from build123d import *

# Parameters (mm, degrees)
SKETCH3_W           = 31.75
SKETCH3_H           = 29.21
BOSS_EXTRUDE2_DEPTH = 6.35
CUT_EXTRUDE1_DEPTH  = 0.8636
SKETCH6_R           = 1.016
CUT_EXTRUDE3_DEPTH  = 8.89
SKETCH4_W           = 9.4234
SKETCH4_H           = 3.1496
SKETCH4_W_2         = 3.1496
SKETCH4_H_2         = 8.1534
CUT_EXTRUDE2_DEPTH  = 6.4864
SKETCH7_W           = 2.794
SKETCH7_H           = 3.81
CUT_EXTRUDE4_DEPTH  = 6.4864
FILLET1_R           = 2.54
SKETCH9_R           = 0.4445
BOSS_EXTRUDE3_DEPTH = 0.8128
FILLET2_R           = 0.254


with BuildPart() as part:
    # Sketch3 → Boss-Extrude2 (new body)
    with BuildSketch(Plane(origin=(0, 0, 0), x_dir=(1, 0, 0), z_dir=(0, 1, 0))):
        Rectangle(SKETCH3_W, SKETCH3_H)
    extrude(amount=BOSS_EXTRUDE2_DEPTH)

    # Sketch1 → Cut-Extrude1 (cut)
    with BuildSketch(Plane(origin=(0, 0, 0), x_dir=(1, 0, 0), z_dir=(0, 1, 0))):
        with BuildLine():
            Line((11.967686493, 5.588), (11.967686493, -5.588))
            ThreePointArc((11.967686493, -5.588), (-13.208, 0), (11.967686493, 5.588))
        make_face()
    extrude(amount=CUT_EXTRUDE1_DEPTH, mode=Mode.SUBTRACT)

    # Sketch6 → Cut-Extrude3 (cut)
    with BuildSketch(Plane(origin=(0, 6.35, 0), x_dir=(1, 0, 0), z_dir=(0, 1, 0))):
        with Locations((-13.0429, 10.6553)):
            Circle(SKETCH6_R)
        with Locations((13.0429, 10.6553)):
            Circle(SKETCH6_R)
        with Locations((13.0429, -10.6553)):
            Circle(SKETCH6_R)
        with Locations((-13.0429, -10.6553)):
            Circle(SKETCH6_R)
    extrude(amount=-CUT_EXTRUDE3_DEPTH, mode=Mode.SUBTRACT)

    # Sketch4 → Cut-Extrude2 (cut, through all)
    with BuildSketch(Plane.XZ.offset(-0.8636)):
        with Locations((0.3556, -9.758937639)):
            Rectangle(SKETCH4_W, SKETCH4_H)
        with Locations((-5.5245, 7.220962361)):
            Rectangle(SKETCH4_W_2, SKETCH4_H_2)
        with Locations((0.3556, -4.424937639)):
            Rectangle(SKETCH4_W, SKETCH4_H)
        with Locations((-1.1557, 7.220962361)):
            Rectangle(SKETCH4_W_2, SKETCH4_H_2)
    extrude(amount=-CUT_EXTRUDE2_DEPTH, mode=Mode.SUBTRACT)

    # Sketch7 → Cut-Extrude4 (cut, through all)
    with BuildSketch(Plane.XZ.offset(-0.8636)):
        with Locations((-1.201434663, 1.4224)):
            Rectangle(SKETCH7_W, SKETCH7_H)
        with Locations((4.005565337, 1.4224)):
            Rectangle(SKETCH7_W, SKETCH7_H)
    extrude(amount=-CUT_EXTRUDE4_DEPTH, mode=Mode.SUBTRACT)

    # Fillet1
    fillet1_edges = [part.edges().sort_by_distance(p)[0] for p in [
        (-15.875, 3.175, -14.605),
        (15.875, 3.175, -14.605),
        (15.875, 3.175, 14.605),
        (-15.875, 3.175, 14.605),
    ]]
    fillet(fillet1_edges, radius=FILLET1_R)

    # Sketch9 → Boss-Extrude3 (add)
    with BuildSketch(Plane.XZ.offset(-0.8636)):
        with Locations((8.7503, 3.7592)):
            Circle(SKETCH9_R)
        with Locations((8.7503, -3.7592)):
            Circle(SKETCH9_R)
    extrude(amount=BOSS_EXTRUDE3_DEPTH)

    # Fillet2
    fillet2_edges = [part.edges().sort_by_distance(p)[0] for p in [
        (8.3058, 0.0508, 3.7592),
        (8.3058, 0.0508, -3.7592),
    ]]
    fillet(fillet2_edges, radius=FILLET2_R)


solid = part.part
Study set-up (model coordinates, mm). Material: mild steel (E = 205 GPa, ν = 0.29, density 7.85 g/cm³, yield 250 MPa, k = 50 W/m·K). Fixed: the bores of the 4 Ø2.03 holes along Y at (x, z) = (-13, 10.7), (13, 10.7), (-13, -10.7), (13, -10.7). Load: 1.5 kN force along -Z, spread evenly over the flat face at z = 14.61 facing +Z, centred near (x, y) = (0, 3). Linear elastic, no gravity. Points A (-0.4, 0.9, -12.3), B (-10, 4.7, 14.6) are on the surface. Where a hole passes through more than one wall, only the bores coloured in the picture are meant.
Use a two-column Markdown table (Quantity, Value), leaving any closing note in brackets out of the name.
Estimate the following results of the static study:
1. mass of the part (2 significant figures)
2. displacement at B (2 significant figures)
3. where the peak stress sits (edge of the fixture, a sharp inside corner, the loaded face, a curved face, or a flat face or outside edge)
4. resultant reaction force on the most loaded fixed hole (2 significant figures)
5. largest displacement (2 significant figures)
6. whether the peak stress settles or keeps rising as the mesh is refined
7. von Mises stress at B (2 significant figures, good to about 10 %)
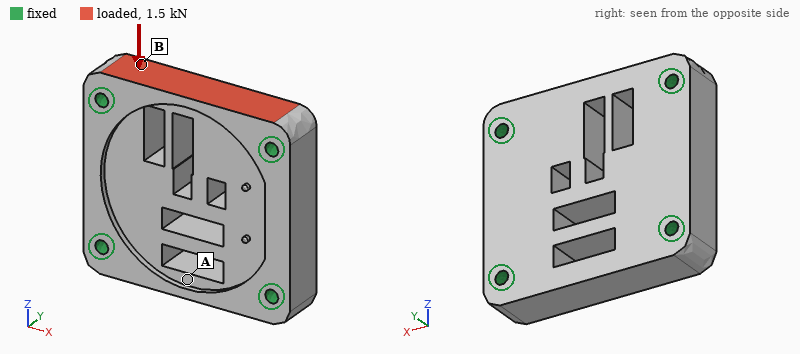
| Quantity | Value |
|---|---|
| mass of the part | 36 g |
| displacement at B | 0.61 µm |
| where the peak stress sits | a sharp inside corner |
| resultant reaction force on the most loaded fixed hole | 530 N |
| largest displacement | 2.3 µm |
| whether the peak stress settles or keeps rising as the mesh is refined | keeps rising |
| von Mises stress at B | 11 MPa |
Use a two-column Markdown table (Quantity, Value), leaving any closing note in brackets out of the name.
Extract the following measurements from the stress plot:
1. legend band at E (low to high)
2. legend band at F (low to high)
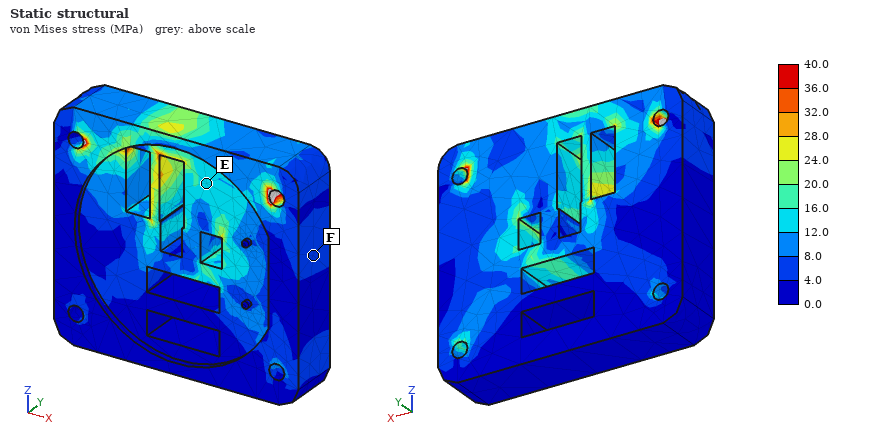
| Quantity | Value |
|---|---|
| legend band at E | 12.0 to 16.0 MPa |
| legend band at F | 4.0 to 8.0 MPa |
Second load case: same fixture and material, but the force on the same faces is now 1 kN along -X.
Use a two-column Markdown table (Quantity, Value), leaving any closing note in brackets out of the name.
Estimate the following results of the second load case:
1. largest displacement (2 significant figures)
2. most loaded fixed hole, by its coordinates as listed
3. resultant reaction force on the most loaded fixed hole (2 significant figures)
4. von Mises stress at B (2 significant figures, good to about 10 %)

| Quantity | Value |
|---|---|
| largest displacement | 0.79 µm |
| most loaded fixed hole, by its coordinates as listed | (13, 10.7) |
| resultant reaction force on the most loaded fixed hole | 560 N |
| von Mises stress at B | 12 MPa |
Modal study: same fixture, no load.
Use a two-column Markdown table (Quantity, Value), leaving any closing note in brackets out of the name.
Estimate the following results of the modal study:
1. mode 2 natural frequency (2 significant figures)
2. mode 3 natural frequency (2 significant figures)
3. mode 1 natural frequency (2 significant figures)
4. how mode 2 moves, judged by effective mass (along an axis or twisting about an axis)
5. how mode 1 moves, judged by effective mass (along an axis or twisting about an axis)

| Quantity | Value |
|---|---|
| mode 2 natural frequency | 39 kHz |
| mode 3 natural frequency | 44 kHz |
| mode 1 natural frequency | 28 kHz |
| how mode 2 moves, judged by effective mass | twisting about X |
| how mode 1 moves, judged by effective mass | along Y |
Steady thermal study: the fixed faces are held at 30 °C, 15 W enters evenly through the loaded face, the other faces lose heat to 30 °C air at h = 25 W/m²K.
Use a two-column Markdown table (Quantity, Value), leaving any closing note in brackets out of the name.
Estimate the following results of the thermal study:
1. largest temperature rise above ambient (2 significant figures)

| Quantity | Value |
|---|---|
| largest temperature rise above ambient | 25 K |
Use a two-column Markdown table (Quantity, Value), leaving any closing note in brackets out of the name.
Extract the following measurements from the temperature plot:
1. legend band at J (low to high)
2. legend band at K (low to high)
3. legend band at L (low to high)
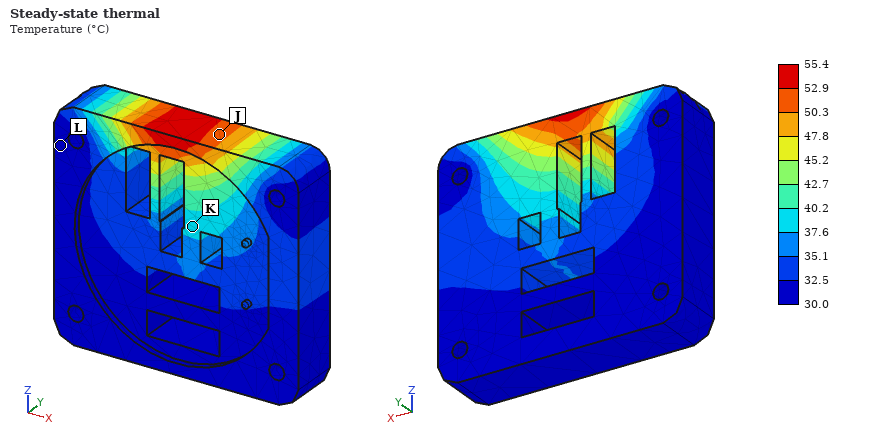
| Quantity | Value |
|---|---|
| legend band at J | 50.3 to 52.9 °C |
| legend band at K | 37.6 to 40.2 °C |
| legend band at L | 30.0 to 32.5 °C |
